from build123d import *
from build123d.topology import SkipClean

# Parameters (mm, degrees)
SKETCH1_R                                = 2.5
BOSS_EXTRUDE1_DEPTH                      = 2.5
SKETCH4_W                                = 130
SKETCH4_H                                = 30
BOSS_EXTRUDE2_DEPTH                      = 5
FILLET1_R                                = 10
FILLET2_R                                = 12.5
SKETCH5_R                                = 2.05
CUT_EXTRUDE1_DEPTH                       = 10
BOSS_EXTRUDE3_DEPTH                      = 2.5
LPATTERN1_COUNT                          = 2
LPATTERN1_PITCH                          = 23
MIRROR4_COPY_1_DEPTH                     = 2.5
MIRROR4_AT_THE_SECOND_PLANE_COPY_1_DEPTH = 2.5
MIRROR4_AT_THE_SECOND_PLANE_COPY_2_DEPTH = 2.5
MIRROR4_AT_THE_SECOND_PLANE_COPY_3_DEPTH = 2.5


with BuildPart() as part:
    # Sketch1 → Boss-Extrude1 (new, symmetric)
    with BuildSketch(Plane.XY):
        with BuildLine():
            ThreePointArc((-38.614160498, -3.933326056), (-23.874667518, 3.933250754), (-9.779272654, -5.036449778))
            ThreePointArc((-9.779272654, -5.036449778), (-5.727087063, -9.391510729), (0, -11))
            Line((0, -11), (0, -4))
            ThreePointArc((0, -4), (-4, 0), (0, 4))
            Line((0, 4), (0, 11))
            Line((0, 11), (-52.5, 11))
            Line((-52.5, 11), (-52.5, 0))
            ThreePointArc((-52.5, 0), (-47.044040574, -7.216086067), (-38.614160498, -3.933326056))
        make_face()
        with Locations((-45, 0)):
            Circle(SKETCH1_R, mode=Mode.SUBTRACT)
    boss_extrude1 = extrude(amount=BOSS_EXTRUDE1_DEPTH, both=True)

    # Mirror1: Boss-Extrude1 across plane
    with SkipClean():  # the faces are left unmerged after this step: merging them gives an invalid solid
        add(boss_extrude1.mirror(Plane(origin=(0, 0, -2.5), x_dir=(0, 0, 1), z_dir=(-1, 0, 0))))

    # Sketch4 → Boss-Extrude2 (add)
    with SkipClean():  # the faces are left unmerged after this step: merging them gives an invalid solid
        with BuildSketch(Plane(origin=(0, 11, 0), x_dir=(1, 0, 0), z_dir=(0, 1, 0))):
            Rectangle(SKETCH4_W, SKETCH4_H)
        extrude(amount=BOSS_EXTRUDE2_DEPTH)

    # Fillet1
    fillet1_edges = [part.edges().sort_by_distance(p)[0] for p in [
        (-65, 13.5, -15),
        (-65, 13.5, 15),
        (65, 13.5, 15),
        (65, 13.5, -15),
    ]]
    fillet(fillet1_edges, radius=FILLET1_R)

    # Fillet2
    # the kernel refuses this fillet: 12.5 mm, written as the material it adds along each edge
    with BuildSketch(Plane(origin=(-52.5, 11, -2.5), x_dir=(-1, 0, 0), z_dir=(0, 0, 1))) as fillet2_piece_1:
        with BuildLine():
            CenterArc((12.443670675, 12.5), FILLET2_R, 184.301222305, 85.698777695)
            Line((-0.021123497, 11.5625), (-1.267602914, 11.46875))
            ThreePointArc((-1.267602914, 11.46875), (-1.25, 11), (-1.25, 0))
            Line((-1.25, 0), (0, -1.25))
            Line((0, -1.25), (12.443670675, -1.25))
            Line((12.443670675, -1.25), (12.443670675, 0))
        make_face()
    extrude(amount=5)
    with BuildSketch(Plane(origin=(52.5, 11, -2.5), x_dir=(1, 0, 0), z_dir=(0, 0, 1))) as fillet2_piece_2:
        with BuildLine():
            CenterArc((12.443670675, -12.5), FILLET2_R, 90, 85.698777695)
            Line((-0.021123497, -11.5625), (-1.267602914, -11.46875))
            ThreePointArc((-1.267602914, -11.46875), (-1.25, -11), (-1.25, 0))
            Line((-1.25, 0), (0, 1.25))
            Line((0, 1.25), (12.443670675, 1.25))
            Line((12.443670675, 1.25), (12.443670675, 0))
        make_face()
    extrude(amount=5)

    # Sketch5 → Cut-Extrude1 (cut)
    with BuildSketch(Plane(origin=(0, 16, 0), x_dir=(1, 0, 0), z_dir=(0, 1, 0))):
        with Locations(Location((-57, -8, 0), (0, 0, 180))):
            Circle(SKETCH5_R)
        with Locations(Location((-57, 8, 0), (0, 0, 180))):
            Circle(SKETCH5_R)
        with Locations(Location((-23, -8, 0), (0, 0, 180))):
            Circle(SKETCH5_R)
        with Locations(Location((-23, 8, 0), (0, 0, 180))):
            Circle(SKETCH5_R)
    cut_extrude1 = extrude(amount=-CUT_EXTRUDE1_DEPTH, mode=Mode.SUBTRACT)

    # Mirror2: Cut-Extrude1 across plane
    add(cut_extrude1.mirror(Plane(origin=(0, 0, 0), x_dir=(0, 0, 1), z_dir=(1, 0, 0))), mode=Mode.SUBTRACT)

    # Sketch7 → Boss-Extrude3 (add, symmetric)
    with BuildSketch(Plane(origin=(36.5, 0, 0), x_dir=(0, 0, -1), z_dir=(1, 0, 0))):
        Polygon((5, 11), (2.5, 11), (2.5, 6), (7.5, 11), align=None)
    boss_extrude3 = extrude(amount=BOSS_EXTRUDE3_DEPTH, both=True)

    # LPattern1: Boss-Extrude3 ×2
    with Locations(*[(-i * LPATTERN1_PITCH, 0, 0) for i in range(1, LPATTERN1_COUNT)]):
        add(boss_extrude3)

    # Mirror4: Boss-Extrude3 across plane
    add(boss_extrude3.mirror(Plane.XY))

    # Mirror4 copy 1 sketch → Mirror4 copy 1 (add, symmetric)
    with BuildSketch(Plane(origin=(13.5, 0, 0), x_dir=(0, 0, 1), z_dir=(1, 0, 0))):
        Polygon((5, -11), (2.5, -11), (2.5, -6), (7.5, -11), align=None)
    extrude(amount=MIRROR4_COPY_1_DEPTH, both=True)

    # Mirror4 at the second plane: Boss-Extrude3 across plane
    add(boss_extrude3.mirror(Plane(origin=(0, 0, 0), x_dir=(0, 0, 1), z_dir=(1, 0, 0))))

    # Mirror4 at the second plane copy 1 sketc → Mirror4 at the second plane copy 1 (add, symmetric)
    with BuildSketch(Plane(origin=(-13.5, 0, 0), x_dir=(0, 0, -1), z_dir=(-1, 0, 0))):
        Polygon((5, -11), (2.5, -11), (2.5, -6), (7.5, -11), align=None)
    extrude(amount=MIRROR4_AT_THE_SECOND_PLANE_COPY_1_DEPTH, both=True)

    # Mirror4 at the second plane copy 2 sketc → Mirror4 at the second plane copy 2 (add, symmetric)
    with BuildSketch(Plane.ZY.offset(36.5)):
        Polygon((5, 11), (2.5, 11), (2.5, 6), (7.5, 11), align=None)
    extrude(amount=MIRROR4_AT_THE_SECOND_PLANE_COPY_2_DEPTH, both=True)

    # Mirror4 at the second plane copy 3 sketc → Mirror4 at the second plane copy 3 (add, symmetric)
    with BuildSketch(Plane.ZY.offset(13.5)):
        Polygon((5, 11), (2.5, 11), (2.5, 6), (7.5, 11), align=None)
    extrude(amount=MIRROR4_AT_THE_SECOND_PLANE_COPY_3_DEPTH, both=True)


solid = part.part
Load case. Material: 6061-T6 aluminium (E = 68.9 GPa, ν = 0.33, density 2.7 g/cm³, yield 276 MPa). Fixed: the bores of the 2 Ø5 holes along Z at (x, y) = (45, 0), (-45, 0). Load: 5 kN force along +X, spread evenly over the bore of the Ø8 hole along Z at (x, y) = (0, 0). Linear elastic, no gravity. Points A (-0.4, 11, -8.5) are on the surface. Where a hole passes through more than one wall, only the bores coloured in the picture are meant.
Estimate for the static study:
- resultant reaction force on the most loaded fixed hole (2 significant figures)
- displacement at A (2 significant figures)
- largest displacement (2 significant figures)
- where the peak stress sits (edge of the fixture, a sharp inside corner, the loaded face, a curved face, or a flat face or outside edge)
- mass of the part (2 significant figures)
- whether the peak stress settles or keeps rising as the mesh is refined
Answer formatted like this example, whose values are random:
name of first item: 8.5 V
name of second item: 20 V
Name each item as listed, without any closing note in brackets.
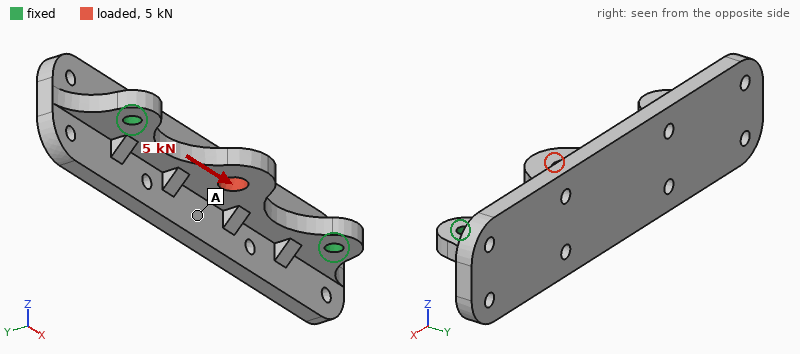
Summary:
resultant reaction force on the most loaded fixed hole: 2.5 kN
displacement at A: 37 µm
largest displacement: 89 µm
where the peak stress sits: edge of the fixture
mass of the part: 70 g
whether the peak stress settles or keeps rising as the mesh is refined: keeps rising
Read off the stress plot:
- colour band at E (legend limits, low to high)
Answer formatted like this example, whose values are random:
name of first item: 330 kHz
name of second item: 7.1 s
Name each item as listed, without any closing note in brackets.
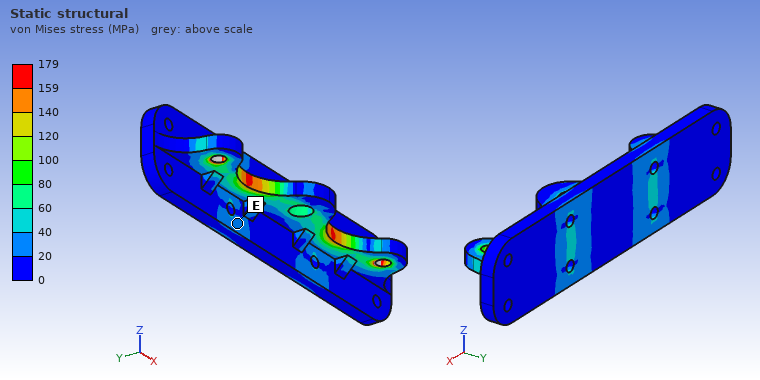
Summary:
colour band at E: 20 to 40 MPa
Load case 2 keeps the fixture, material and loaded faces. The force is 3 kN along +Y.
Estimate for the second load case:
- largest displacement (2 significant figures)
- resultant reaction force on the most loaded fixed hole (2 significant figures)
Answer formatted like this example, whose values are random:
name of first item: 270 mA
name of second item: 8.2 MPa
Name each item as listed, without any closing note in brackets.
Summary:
largest displacement: 76 µm
resultant reaction force on the most loaded fixed hole: 2.5 kN
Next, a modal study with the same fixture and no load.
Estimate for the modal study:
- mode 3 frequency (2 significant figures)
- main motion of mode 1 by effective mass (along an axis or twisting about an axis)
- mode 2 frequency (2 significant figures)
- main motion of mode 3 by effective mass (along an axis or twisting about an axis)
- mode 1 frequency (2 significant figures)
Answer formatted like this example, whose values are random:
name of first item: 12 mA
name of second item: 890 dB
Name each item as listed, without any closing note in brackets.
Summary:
mode 3 frequency: 5300 Hz
main motion of mode 1 by effective mass: along Z
mode 2 frequency: 5000 Hz
main motion of mode 3 by effective mass: along Z
mode 1 frequency: 3000 Hz
